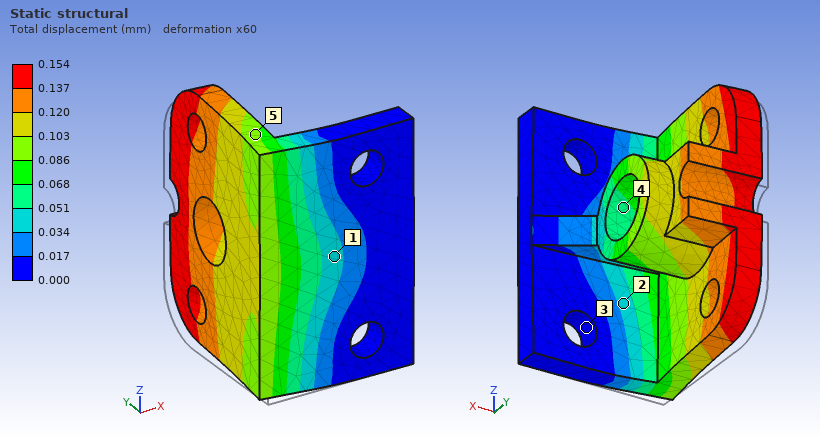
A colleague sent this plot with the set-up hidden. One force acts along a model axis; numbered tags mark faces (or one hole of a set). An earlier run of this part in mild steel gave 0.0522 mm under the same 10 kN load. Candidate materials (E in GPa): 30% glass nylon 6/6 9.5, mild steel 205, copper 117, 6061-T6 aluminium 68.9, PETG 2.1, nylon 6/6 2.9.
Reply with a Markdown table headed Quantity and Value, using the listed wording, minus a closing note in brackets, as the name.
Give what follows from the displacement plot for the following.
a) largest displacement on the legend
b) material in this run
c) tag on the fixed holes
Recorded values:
| Quantity | Value |
|---|---|
| largest displacement on the legend | 0.154 mm |
| material in this run | 6061-T6 aluminium |
| tag on the fixed holes | 3 |
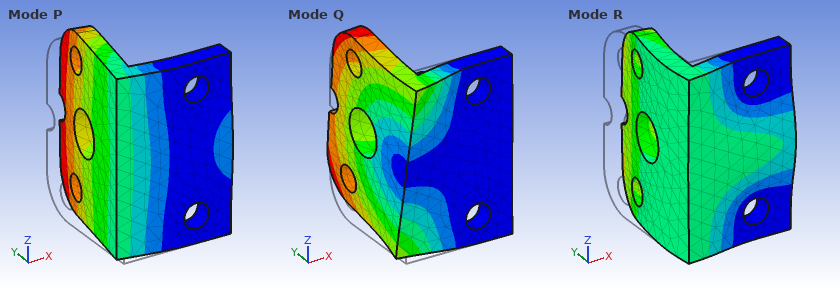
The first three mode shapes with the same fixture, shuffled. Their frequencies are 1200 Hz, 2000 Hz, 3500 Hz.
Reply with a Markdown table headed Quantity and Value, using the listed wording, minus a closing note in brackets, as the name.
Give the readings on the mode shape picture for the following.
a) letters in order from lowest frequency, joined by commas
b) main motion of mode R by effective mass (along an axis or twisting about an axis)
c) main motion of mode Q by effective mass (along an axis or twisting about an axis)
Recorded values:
| Quantity | Value |
|---|---|
| letters in order from lowest frequency, joined by commas | P, Q, R |
| main motion of mode R by effective mass | along Y |
| main motion of mode Q by effective mass | along Z |
